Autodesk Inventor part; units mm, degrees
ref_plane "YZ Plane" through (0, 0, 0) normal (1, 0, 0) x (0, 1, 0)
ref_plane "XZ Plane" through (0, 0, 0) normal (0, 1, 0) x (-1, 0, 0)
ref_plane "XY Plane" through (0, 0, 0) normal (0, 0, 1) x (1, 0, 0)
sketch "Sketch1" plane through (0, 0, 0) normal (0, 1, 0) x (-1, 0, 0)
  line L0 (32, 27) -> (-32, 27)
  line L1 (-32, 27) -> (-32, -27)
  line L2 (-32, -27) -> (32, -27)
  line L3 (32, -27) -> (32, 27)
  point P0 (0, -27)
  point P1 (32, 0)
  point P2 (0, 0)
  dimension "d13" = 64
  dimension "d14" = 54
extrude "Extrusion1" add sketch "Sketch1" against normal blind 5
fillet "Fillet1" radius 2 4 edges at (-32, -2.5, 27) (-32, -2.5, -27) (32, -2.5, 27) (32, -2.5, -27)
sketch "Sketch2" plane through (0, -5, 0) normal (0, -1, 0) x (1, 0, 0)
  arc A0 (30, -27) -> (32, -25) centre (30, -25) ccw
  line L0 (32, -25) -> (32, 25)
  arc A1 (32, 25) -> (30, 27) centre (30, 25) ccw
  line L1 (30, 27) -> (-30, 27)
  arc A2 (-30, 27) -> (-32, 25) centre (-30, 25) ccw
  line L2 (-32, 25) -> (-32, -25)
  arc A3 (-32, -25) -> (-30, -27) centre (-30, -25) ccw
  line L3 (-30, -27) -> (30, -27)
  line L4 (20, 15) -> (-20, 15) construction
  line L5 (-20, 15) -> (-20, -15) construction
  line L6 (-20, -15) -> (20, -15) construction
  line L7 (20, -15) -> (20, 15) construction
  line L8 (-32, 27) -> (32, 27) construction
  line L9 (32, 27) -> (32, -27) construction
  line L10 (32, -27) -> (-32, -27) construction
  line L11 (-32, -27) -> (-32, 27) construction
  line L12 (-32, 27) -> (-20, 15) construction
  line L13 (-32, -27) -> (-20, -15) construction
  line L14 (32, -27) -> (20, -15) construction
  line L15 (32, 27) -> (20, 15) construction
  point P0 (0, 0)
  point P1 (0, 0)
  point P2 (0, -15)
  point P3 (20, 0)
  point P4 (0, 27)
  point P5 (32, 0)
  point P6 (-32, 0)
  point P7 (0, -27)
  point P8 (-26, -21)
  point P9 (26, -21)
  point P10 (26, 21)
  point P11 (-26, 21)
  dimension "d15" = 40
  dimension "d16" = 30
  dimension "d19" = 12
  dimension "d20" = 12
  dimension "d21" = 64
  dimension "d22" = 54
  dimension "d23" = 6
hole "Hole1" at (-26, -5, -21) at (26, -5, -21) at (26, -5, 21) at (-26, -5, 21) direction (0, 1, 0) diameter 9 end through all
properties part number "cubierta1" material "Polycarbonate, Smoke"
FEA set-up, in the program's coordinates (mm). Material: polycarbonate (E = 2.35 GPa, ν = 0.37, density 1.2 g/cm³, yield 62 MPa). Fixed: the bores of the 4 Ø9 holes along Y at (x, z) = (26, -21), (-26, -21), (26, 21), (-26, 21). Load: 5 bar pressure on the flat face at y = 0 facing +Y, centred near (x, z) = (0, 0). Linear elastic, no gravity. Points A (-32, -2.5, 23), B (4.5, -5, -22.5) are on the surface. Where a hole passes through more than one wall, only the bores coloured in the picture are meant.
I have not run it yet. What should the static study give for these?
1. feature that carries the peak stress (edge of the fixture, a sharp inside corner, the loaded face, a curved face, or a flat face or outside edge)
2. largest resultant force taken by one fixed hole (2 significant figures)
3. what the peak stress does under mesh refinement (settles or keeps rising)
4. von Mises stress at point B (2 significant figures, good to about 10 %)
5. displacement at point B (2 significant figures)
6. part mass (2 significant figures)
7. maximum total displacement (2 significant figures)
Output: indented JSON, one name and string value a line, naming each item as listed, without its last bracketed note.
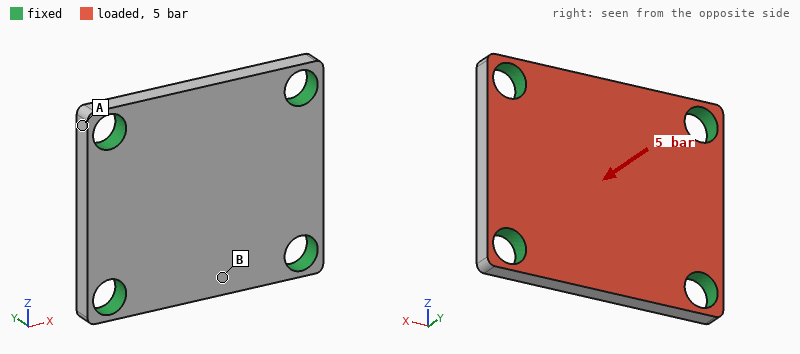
{
  "feature that carries the peak stress": "edge of the fixture",
  "largest resultant force taken by one fixed hole": "400 N",
  "what the peak stress does under mesh refinement": "keeps rising",
  "von Mises stress at point B": "11 MPa",
  "displacement at point B": "0.28 mm",
  "part mass": "19 g",
  "maximum total displacement": "0.44 mm"
}
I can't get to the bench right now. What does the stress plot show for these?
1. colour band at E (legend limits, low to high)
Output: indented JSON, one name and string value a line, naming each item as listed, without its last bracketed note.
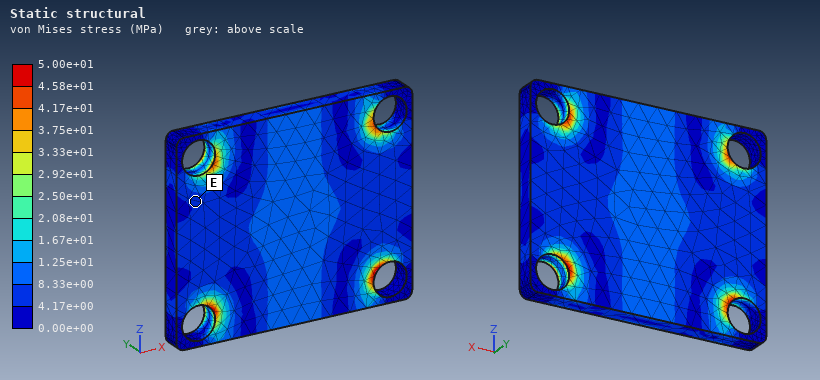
{
  "colour band at E": "4.17e+00 to 8.33e+00 MPa"
}
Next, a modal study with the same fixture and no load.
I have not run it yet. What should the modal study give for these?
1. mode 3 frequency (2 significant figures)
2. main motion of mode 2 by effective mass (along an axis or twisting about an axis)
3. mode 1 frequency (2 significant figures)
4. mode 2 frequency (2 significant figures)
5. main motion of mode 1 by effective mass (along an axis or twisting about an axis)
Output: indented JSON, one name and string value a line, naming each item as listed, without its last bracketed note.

{
  "mode 3 frequency": "4600 Hz",
  "main motion of mode 2 by effective mass": "twisting about X",
  "mode 1 frequency": "2600 Hz",
  "mode 2 frequency": "3700 Hz",
  "main motion of mode 1 by effective mass": "along Y"
}
